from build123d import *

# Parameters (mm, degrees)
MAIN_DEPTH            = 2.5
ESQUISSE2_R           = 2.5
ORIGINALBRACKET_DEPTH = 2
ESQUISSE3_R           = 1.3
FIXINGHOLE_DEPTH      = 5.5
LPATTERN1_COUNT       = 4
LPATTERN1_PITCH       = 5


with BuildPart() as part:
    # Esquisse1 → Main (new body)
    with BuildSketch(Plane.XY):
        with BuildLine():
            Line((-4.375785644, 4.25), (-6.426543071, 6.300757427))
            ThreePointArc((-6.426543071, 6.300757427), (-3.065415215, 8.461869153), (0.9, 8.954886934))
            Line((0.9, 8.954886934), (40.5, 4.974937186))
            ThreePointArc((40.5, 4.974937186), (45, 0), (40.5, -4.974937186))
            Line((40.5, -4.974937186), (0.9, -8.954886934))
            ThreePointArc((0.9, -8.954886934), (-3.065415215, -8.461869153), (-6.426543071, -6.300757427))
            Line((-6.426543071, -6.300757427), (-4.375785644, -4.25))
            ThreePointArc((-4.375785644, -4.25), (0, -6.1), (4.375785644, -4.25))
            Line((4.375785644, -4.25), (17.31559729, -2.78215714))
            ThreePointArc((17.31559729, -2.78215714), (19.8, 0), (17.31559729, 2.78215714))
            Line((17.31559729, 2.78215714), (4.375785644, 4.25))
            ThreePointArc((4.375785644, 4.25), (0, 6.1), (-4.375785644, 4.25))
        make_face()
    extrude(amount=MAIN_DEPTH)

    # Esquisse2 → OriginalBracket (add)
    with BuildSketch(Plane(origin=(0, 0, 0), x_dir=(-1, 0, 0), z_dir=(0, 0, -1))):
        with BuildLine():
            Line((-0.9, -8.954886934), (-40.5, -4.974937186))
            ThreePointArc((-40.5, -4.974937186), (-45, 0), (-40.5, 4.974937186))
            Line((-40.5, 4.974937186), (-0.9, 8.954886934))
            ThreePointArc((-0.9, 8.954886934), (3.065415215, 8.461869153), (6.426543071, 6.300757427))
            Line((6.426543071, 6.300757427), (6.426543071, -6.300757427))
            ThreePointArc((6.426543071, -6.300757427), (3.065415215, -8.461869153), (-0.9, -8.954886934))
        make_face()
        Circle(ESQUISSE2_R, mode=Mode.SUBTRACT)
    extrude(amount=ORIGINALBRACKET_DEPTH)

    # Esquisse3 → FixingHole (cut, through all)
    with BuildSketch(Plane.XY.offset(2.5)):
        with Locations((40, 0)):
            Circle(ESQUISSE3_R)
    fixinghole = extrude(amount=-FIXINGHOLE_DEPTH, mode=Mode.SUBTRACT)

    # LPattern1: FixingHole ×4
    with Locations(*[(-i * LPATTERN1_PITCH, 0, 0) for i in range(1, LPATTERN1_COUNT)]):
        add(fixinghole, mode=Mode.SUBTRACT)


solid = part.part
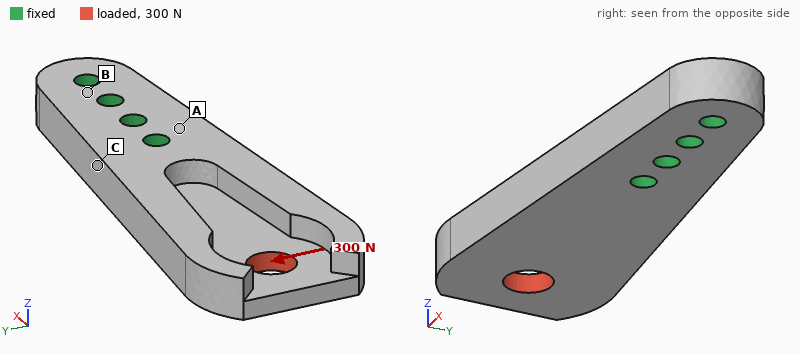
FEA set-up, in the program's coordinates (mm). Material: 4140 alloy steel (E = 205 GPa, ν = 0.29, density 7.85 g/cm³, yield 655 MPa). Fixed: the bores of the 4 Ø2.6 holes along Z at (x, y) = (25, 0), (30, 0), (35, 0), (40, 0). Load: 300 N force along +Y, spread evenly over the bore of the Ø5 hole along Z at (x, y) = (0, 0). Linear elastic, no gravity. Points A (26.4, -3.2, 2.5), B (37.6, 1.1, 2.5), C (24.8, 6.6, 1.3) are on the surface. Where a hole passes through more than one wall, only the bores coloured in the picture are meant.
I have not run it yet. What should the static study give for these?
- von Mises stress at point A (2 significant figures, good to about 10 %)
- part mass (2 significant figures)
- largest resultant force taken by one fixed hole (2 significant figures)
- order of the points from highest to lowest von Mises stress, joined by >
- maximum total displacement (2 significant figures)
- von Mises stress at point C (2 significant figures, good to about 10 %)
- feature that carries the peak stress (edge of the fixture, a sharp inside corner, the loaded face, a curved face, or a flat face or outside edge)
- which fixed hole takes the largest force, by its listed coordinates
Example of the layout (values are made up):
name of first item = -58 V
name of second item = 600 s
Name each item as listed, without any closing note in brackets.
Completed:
von Mises stress at point A = 34 MPa
part mass = 20 g
largest resultant force taken by one fixed hole = 910 N
order of the points from highest to lowest von Mises stress, joined by > = C > A > B
maximum total displacement = 24 µm
von Mises stress at point C = 55 MPa
feature that carries the peak stress = edge of the fixture
which fixed hole takes the largest force, by its listed coordinates = (25, 0)
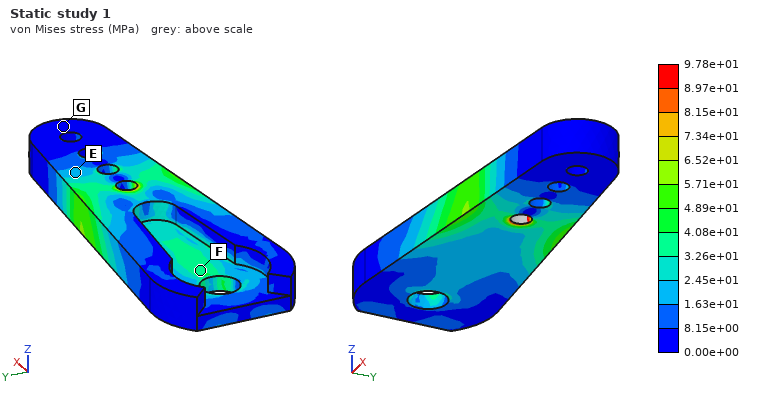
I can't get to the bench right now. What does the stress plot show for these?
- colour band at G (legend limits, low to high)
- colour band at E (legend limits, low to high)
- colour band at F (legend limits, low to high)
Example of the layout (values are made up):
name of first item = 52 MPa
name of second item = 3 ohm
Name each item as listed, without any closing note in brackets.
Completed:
colour band at G = 0.00e+00 to 8.15e+00 MPa
colour band at E = 1.63e+01 to 2.45e+01 MPa
colour band at F = 3.26e+01 to 4.08e+01 MPa
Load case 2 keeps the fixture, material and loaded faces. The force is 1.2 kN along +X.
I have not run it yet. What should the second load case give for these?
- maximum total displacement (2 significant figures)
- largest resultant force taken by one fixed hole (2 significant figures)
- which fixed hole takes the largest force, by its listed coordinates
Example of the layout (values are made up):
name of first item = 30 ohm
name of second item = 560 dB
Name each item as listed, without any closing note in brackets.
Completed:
maximum total displacement = 31 µm
largest resultant force taken by one fixed hole = 840 N
which fixed hole takes the largest force, by its listed coordinates = (25, 0)
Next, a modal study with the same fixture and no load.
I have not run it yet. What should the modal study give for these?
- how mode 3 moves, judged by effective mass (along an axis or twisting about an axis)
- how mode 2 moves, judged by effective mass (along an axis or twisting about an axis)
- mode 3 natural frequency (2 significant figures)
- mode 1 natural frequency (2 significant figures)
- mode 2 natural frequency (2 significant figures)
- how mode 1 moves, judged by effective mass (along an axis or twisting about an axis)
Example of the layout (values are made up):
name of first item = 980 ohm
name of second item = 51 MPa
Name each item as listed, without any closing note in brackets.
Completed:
how mode 3 moves, judged by effective mass = along Y
how mode 2 moves, judged by effective mass = along Y
mode 3 natural frequency = 9400 Hz
mode 1 natural frequency = 3900 Hz
mode 2 natural frequency = 7800 Hz
how mode 1 moves, judged by effective mass = along Z
